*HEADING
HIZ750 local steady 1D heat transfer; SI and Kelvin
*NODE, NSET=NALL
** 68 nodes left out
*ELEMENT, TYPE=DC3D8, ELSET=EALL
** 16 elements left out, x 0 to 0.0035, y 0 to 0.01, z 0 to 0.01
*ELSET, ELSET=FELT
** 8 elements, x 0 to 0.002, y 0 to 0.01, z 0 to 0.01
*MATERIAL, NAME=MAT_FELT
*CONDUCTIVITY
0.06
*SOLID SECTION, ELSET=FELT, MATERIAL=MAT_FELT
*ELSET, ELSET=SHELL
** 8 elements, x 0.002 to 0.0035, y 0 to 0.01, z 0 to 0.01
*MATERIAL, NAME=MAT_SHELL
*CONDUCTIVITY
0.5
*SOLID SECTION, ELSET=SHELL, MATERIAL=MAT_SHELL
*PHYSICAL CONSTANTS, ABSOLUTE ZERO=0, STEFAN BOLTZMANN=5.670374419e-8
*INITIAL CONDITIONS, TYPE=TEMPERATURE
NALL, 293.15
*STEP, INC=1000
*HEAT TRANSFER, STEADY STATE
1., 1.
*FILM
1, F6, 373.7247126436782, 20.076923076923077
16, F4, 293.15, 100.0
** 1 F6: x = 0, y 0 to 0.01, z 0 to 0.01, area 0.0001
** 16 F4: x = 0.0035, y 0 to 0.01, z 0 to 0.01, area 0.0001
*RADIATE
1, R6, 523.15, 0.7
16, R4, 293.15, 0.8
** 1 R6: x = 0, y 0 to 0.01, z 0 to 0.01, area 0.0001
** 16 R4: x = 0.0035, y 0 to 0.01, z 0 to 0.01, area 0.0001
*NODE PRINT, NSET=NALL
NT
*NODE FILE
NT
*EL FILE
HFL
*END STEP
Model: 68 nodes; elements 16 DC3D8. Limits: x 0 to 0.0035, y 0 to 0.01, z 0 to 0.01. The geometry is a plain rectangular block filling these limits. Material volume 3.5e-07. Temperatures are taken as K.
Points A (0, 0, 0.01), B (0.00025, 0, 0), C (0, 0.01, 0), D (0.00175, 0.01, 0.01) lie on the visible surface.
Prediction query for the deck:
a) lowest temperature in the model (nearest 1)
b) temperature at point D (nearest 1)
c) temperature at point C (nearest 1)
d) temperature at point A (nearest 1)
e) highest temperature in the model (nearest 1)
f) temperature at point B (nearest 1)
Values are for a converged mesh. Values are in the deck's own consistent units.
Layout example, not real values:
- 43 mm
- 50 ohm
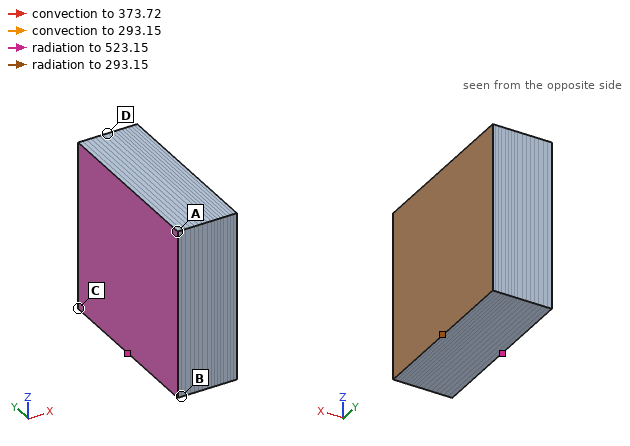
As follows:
- 312 K
- 326 K
- 382 K
- 382 K
- 382 K
- 374 K
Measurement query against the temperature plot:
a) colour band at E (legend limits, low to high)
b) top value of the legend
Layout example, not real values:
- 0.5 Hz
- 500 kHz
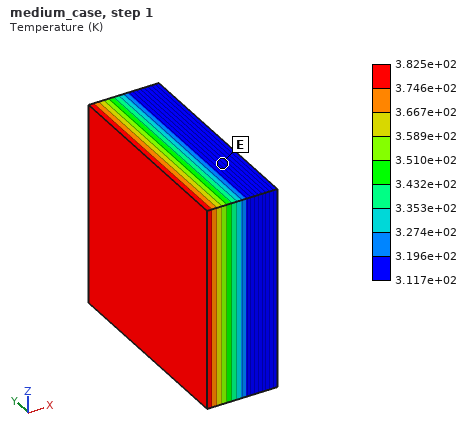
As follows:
- 3.117e+02 to 3.196e+02 K
- 3.825e+02 K
